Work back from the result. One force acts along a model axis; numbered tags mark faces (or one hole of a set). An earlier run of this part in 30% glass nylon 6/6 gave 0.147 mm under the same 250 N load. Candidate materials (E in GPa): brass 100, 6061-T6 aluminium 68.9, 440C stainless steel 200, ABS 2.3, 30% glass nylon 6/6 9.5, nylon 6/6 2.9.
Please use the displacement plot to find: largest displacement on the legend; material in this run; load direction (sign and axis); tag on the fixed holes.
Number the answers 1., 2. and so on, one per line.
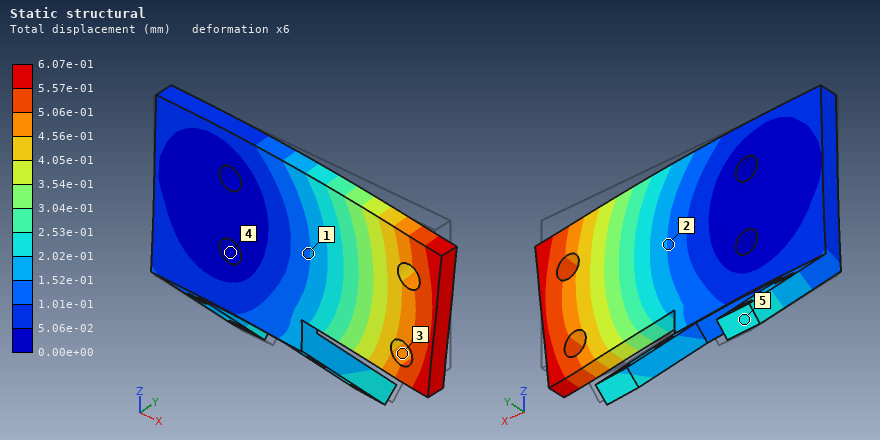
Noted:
1. 6.07e-01 mm
2. ABS
3. -Z
4. 4
